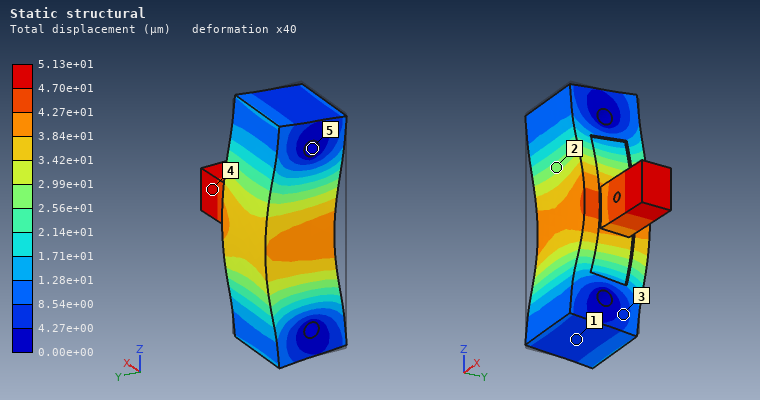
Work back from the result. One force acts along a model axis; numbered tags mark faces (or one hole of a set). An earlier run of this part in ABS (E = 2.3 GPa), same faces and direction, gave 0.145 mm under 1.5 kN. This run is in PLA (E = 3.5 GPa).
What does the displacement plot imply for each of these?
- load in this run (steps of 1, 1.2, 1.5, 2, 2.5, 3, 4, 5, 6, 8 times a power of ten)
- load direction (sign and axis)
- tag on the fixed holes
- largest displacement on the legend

800 N
+Y
5
5.13e+01 µm
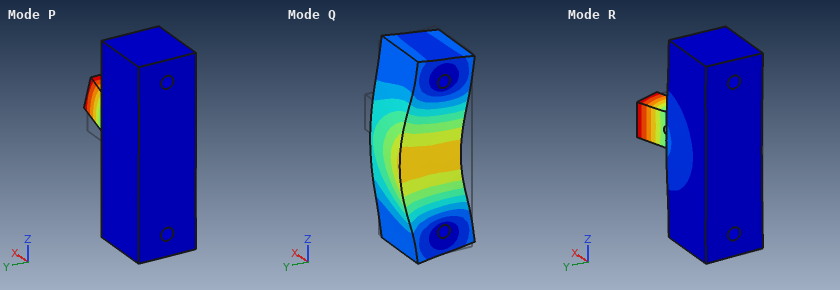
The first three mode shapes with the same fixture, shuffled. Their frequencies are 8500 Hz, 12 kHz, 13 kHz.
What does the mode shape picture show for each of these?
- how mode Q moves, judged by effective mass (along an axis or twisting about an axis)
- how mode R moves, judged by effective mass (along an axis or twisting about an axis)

along Y
along Y
